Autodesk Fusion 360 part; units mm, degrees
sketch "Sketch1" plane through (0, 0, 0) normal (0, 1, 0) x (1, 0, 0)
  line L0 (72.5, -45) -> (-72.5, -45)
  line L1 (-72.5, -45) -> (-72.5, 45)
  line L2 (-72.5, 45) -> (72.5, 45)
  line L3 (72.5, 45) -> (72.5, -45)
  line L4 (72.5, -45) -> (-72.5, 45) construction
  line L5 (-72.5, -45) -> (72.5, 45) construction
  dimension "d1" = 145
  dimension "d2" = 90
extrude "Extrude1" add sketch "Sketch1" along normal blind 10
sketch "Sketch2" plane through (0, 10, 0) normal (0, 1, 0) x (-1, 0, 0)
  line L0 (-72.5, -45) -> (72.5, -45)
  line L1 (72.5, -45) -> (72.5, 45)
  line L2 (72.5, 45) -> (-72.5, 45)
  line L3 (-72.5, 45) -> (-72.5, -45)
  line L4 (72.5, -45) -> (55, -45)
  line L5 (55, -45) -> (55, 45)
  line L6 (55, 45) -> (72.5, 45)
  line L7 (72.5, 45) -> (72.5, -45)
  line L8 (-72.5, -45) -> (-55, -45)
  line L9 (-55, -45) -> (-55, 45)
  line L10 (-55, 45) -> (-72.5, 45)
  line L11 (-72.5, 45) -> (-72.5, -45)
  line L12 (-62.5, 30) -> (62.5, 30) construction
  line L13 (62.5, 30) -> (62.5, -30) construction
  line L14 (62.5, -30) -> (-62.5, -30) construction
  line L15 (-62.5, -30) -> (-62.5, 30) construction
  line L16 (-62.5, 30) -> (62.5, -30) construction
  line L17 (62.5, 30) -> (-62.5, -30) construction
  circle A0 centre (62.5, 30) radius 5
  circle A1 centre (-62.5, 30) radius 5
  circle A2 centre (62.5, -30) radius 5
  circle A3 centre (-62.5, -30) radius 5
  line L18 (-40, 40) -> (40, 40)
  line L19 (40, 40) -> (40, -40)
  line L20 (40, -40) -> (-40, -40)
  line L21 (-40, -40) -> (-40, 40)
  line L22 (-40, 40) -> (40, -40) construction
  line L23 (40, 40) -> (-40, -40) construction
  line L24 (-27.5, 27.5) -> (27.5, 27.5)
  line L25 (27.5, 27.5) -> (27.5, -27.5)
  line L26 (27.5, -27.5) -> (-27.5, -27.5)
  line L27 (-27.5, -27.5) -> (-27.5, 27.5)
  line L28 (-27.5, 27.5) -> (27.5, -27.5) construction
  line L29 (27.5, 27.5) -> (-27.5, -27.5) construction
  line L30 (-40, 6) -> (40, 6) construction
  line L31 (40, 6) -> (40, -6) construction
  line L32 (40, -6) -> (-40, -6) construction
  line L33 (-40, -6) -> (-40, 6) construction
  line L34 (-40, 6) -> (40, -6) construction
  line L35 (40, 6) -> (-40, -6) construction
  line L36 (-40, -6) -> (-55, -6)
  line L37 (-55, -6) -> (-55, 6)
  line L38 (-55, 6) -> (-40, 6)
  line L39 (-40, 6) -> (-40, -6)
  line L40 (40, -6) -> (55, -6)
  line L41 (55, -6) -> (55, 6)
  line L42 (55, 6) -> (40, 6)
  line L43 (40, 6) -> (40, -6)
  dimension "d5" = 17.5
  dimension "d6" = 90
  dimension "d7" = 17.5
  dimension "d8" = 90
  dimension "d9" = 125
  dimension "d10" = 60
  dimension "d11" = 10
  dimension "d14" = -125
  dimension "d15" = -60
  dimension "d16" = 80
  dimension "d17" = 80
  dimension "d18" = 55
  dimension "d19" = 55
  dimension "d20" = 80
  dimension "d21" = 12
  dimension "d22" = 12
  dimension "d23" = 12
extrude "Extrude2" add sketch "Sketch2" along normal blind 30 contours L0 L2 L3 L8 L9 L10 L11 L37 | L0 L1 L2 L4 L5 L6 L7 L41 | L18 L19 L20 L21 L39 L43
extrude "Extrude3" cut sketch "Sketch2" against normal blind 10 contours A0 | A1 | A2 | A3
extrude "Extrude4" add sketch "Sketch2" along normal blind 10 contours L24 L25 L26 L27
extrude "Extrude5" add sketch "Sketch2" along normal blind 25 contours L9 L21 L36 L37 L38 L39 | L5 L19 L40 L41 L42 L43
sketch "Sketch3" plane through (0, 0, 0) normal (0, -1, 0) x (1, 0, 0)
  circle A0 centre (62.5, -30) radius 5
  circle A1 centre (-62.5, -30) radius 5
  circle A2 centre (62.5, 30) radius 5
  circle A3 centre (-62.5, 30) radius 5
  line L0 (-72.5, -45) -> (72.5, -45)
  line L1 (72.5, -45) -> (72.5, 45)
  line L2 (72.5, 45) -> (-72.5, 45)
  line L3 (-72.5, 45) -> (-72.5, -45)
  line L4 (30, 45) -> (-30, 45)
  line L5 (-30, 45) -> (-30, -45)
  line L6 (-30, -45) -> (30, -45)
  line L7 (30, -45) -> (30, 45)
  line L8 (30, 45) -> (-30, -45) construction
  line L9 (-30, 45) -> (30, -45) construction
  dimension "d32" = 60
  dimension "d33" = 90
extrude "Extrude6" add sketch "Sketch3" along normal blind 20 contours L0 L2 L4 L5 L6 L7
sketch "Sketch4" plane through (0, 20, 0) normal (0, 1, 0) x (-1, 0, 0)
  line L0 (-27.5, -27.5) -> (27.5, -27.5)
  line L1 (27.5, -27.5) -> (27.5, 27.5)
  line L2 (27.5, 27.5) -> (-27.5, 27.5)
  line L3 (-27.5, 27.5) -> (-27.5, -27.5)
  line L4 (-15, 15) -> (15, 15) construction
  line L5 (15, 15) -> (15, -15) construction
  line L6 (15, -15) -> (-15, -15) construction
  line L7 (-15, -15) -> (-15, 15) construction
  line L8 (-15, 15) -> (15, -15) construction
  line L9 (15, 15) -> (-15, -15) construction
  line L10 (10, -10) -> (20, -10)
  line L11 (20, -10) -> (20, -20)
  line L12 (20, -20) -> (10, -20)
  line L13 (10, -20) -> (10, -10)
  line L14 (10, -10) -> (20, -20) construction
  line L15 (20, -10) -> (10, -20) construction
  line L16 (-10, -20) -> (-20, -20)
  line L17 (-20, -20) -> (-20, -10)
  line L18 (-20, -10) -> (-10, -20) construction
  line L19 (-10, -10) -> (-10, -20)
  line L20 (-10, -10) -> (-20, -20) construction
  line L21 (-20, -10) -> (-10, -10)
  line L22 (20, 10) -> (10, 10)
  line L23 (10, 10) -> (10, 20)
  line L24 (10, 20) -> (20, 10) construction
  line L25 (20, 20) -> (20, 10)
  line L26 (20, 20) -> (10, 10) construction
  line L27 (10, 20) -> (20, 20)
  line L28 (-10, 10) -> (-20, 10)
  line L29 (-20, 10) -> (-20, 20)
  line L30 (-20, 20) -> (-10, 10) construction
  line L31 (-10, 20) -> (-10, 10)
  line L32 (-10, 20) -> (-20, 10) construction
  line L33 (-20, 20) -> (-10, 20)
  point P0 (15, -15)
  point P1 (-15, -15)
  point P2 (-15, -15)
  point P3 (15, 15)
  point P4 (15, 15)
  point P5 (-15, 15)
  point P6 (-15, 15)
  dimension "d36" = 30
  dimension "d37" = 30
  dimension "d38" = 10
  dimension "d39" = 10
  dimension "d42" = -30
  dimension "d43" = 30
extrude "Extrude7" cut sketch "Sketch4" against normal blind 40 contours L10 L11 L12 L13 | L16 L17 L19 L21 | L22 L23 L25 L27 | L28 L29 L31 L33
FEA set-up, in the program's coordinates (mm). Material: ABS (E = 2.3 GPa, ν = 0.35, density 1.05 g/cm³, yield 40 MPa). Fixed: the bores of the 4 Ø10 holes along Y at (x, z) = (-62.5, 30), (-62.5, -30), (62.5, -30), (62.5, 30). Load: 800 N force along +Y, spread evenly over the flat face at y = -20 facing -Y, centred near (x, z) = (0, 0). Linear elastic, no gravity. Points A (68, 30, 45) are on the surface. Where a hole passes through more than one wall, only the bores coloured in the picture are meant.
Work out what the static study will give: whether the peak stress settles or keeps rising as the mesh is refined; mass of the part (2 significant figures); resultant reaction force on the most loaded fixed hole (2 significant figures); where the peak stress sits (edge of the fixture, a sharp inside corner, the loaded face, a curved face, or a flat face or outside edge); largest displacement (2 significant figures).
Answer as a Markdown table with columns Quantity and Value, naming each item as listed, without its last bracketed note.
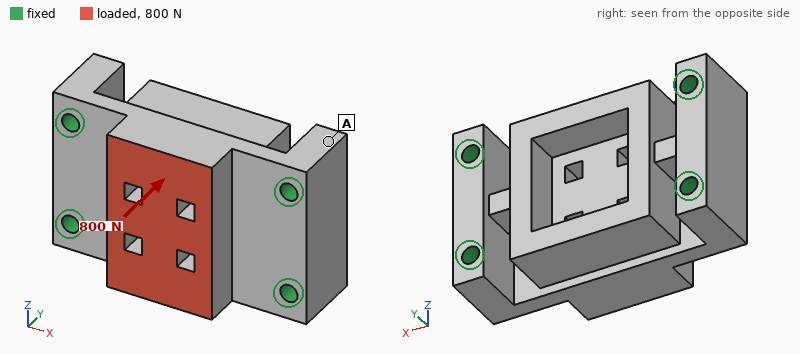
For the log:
| Quantity | Value |
|---|---|
| whether the peak stress settles or keeps rising as the mesh is refined | keeps rising |
| mass of the part | 470 g |
| resultant reaction force on the most loaded fixed hole | 200 N |
| where the peak stress sits | edge of the fixture |
| largest displacement | 45 µm |
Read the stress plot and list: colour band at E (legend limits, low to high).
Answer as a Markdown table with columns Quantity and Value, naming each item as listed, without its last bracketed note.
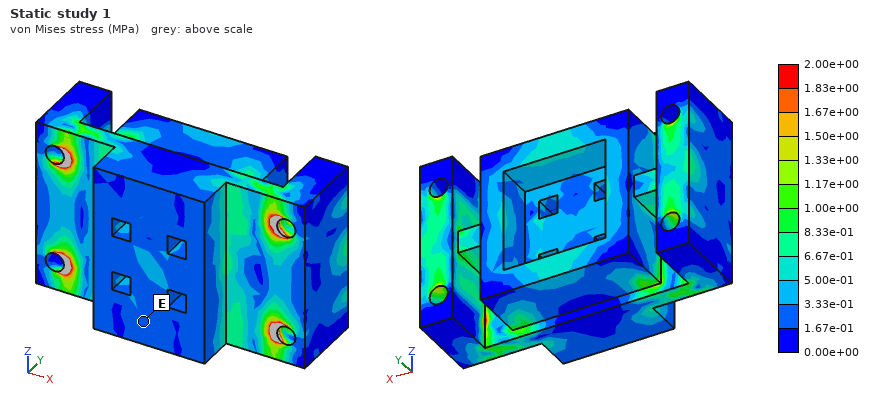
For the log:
| Quantity | Value |
|---|---|
| colour band at E | 1.67e-01 to 3.33e-01 MPa |
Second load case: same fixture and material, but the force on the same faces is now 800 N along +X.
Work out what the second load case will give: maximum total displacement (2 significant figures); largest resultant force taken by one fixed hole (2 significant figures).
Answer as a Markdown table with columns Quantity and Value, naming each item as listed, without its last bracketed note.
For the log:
| Quantity | Value |
|---|---|
| maximum total displacement | 31 µm |
| largest resultant force taken by one fixed hole | 230 N |
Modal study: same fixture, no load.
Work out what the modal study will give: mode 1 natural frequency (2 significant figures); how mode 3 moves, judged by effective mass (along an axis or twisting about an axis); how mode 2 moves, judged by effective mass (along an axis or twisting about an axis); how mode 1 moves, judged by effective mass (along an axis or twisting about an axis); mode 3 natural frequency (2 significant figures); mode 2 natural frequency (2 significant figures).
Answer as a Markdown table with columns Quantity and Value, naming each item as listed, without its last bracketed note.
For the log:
| Quantity | Value |
|---|---|
| mode 1 natural frequency | 1200 Hz |
| how mode 3 moves, judged by effective mass | along Z |
| how mode 2 moves, judged by effective mass | along Y |
| how mode 1 moves, judged by effective mass | twisting about X |
| mode 3 natural frequency | 1900 Hz |
| mode 2 natural frequency | 1300 Hz |
